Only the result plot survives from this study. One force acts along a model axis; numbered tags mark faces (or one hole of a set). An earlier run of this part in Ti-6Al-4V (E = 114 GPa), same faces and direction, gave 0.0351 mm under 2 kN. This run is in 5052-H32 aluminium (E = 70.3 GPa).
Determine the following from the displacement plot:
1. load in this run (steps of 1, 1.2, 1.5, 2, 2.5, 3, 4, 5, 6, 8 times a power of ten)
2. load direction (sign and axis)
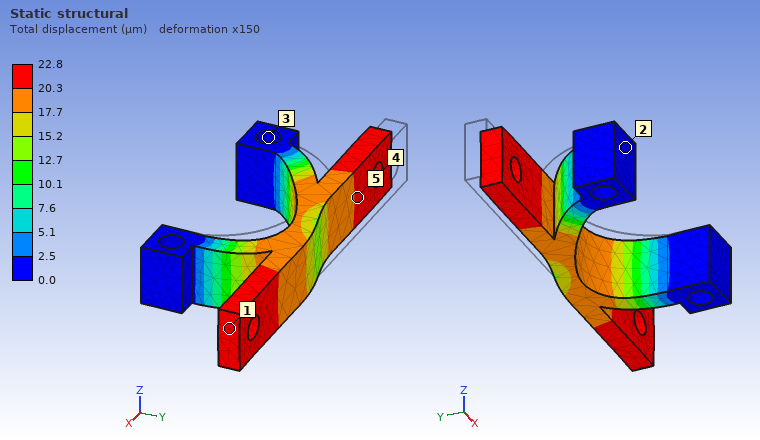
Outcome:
800 N
+X
